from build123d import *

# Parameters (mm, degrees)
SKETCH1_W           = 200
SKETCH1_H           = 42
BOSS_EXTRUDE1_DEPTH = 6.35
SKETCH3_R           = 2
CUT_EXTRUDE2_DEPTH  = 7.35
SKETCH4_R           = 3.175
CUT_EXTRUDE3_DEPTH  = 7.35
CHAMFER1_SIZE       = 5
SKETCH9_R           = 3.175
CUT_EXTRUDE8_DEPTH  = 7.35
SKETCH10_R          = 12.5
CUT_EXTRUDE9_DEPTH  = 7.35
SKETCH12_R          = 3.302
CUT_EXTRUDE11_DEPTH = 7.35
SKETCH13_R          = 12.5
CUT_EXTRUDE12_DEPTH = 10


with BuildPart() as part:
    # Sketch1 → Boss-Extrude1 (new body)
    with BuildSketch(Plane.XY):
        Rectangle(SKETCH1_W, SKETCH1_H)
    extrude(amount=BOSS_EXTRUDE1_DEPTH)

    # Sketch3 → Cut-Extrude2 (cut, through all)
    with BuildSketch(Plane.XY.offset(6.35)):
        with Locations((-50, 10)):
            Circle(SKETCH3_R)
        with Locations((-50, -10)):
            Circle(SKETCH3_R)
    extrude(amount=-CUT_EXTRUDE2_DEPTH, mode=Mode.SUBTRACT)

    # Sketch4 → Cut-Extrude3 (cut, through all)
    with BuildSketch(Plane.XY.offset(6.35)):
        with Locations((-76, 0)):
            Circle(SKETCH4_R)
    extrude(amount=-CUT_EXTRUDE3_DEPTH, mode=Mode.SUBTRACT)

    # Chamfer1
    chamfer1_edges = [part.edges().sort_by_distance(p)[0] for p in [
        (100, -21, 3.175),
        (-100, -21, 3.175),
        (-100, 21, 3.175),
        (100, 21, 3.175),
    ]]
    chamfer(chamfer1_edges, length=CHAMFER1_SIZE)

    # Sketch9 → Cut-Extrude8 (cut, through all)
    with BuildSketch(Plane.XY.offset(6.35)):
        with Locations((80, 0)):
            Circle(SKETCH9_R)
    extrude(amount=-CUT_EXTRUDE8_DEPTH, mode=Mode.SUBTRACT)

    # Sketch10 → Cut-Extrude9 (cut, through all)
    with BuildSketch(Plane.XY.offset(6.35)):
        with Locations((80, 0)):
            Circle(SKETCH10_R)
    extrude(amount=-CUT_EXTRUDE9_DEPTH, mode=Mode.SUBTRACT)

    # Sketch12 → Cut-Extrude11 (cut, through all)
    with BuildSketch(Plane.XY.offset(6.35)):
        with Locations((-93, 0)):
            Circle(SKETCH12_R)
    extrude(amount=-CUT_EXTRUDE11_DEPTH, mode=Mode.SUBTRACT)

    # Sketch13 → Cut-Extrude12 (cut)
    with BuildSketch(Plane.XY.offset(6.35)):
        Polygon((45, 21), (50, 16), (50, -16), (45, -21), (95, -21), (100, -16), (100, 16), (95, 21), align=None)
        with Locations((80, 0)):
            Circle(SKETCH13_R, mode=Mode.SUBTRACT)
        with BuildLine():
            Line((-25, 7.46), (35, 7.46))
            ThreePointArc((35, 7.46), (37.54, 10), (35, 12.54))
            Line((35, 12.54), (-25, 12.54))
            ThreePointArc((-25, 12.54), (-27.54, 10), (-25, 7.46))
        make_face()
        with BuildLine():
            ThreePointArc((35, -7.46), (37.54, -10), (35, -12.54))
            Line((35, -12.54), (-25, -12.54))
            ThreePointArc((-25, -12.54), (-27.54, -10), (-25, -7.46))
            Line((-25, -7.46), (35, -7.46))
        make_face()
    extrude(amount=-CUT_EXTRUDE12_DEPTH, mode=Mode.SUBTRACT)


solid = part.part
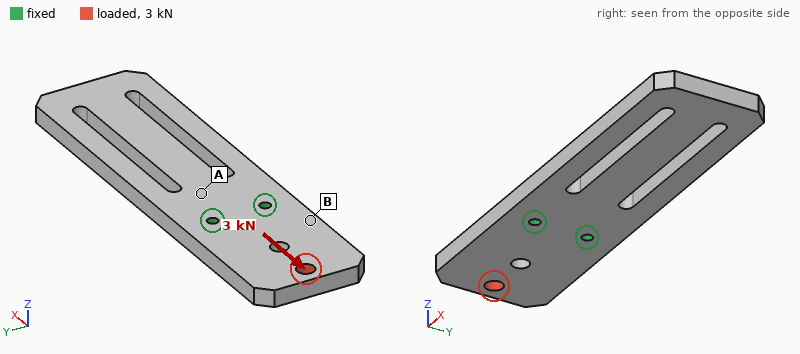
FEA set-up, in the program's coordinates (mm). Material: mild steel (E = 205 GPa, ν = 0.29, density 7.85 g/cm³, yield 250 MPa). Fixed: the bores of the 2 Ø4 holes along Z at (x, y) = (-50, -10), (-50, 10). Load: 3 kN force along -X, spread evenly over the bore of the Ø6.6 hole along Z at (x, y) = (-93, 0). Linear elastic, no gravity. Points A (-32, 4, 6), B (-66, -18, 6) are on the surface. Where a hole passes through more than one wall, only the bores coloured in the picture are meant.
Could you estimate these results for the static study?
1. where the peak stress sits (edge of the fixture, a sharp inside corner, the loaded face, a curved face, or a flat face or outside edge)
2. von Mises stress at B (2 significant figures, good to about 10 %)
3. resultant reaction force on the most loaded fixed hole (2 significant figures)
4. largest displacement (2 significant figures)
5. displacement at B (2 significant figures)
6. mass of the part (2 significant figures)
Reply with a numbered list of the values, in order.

1. the loaded face
2. 9.9 MPa
3. 1.5 kN
4. 5.2 µm
5. 1.3 µm
6. 270 g
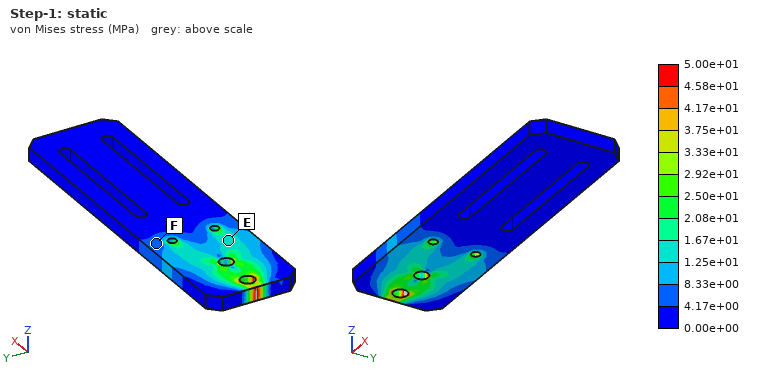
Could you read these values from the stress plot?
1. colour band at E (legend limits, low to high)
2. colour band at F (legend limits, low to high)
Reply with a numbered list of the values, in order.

1. 1.25e+01 to 1.67e+01 MPa
2. 4.17e+00 to 8.33e+00 MPa
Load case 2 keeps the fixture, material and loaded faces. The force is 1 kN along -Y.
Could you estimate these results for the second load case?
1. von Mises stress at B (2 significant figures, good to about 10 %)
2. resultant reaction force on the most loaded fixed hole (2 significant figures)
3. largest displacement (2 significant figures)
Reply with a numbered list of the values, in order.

1. 12 MPa
2. 2.0 kN
3. 9.9 µm
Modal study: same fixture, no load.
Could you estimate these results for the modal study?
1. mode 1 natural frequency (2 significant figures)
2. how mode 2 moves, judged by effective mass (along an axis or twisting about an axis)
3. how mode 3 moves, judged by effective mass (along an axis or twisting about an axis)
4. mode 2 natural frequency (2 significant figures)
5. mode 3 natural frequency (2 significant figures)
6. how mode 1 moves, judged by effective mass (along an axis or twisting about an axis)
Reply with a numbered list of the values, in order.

1. 530 Hz
2. along Y
3. along Z
4. 2000 Hz
5. 2100 Hz
6. along Z
